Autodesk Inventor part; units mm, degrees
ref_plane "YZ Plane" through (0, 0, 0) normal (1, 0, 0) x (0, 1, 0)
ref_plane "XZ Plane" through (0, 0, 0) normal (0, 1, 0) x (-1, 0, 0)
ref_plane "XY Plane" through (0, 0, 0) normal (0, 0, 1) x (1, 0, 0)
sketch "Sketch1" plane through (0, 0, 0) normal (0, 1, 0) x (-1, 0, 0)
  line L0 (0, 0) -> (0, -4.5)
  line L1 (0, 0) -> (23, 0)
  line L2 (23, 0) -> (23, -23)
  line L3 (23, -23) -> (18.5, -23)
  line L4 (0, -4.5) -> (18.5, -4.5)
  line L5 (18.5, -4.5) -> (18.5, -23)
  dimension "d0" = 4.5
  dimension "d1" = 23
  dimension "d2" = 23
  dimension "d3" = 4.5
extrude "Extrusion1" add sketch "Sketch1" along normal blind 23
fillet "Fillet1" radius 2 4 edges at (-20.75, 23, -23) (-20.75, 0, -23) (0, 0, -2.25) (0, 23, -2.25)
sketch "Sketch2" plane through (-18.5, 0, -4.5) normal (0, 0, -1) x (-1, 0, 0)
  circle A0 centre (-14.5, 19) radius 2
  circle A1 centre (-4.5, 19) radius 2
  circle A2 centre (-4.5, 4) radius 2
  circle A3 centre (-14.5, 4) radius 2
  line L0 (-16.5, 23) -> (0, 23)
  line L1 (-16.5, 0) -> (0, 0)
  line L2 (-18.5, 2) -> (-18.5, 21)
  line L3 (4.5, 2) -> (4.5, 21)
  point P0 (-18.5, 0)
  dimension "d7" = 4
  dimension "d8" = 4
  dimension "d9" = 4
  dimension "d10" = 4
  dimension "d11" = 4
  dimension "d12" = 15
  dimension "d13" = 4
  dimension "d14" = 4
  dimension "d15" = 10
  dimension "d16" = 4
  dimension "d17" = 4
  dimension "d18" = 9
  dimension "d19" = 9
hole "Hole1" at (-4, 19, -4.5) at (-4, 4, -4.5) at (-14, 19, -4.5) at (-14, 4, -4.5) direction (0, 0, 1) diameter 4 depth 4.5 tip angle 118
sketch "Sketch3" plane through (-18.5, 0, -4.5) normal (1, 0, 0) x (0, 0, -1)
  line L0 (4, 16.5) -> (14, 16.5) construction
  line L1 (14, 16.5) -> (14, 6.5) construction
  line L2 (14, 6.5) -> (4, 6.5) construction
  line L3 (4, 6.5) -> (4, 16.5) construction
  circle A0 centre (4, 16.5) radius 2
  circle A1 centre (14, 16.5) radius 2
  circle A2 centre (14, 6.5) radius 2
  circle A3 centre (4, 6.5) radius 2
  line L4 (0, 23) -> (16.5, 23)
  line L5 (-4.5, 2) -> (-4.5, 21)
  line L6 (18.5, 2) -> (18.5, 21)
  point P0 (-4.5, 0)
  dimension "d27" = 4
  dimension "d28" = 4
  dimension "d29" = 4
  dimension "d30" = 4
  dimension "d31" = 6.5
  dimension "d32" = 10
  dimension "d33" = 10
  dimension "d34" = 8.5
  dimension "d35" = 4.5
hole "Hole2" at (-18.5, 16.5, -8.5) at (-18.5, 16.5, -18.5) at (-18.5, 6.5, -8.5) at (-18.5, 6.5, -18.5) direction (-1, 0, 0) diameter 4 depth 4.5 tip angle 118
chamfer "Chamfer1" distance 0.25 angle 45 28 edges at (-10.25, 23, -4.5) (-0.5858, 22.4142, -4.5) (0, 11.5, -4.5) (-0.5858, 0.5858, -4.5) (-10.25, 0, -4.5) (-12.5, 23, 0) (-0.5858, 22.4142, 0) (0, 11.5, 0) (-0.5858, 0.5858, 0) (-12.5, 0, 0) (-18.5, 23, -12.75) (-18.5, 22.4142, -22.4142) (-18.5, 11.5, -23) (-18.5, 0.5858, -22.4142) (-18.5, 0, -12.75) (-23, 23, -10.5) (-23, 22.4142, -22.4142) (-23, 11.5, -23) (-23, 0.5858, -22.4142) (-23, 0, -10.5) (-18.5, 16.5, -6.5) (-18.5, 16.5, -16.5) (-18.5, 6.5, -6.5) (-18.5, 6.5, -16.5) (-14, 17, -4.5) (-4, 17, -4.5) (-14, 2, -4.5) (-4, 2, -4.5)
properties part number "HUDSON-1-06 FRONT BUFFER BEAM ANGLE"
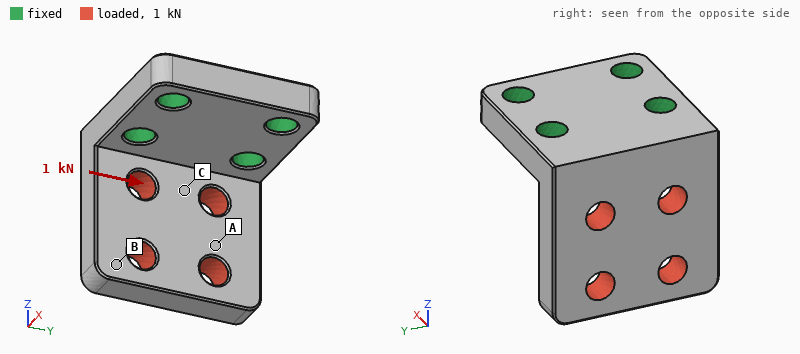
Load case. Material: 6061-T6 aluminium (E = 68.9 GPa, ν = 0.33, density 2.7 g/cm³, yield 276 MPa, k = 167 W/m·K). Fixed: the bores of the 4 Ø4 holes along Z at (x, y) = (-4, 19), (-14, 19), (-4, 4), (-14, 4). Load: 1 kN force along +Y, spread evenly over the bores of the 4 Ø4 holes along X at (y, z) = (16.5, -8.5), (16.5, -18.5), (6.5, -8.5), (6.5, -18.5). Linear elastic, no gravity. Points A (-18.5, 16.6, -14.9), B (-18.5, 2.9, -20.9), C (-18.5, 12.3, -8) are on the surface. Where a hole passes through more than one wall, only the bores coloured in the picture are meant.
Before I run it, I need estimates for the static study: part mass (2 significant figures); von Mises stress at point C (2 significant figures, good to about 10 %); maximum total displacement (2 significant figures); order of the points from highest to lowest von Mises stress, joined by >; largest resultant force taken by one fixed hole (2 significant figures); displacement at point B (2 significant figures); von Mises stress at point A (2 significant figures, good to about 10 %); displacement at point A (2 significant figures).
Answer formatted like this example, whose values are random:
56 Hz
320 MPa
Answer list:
10 g
44 MPa
35 µm
C > A > B
890 N
32 µm
23 MPa
23 µm
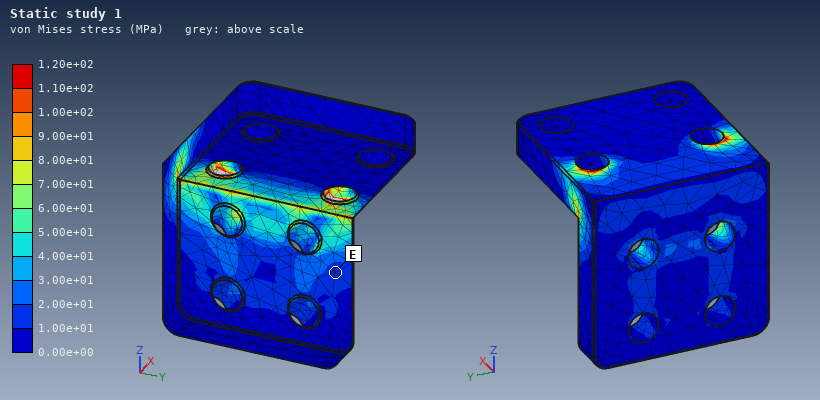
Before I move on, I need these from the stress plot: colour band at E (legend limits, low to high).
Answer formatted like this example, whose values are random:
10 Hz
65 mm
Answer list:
1.00e+01 to 2.00e+01 MPa
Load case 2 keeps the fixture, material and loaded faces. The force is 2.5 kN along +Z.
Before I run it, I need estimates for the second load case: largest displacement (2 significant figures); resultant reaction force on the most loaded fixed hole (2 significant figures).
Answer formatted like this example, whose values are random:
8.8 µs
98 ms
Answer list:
0.10 mm
1.4 kN
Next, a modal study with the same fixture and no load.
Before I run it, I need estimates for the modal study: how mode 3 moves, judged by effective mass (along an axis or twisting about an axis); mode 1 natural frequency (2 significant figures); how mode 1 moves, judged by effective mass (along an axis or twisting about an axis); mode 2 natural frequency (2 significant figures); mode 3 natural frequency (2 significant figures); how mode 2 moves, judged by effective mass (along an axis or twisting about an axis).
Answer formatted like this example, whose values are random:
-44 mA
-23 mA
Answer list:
along Y
6200 Hz
along X
13 kHz
17 kHz
along Y
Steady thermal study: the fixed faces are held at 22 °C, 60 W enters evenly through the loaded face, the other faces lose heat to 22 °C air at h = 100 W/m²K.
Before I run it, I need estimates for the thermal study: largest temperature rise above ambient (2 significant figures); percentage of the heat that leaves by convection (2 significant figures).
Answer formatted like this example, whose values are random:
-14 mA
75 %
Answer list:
60 K
8.6 %
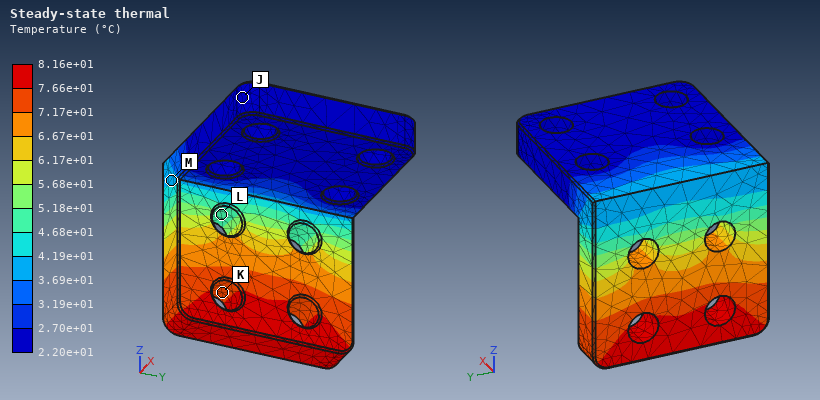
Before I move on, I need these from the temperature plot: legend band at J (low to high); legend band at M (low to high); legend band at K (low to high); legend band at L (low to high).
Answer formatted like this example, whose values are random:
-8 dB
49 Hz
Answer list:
2.20e+01 to 2.70e+01 °C
3.69e+01 to 4.19e+01 °C
7.17e+01 to 7.66e+01 °C
4.68e+01 to 5.18e+01 °C
